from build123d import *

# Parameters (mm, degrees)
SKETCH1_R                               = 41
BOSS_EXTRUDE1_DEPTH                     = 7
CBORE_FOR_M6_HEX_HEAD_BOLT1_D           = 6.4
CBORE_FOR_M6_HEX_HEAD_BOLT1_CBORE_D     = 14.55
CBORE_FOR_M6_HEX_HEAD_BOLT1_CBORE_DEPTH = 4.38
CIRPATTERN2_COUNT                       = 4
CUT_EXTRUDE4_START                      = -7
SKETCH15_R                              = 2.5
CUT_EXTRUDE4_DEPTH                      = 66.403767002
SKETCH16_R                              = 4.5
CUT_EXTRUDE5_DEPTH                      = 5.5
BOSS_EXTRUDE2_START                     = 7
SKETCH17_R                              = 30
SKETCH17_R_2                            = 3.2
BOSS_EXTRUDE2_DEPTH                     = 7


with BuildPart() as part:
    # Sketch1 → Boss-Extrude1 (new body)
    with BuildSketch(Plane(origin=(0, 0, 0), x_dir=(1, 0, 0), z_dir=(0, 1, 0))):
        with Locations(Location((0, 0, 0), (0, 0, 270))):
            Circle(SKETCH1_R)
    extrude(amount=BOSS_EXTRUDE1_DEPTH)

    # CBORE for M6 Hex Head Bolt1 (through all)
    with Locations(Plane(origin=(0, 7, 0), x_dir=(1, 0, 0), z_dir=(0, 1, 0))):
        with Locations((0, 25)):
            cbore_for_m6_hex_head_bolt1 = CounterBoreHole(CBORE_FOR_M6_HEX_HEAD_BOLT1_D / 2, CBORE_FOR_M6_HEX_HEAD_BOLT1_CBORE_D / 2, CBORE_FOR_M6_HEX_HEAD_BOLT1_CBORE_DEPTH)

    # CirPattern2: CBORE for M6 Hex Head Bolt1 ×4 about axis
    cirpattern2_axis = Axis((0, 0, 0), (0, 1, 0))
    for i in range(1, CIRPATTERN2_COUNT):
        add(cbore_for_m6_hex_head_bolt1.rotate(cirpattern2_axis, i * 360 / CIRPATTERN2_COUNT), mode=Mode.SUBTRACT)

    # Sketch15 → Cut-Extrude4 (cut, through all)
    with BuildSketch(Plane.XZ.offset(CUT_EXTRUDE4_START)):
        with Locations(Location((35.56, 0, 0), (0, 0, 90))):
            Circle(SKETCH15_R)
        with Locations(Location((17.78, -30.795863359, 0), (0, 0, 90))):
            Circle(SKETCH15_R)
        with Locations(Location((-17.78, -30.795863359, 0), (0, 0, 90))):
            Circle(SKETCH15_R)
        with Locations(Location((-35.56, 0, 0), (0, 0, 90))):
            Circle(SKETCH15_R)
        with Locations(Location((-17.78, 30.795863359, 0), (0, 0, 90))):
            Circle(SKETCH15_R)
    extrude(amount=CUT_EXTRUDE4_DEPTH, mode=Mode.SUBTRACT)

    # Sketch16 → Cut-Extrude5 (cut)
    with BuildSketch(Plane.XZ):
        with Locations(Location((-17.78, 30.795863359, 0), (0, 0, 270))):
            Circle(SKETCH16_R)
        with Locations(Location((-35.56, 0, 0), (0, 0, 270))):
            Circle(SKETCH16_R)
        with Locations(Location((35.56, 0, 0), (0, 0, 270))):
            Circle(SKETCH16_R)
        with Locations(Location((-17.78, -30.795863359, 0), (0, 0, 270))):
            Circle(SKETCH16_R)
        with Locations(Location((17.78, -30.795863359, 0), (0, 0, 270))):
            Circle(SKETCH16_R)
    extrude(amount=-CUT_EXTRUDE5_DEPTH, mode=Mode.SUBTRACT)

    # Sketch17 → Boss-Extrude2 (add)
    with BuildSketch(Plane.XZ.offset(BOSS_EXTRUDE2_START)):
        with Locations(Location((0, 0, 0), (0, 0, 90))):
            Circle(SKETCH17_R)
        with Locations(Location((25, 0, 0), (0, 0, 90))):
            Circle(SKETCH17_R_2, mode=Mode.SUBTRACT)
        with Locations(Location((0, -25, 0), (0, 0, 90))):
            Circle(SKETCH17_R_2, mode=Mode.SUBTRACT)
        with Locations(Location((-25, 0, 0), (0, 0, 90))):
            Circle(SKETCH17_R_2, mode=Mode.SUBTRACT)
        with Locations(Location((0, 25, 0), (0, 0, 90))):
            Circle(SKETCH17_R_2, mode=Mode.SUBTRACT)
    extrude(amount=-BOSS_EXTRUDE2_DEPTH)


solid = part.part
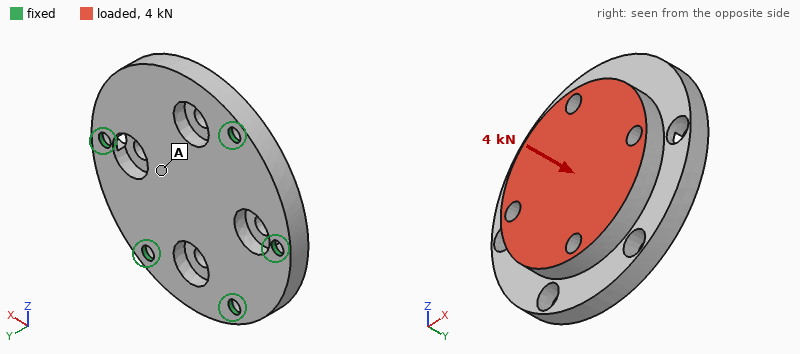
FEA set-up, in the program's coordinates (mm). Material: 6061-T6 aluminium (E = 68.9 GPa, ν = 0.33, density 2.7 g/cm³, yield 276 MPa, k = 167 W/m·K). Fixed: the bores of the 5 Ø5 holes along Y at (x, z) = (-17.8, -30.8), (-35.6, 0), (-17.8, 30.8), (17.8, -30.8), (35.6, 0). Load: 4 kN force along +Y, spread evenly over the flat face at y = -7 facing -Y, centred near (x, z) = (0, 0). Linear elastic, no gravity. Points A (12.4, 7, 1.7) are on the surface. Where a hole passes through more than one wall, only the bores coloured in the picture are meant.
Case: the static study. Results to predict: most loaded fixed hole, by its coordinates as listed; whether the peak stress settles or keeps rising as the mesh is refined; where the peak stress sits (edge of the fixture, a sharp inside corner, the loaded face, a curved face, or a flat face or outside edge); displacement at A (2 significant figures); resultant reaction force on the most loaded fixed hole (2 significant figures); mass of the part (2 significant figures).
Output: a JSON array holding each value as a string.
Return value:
["(-17.8, 30.8)", "keeps rising", "edge of the fixture", "22 µm", "1.7 kN", "140 g"]
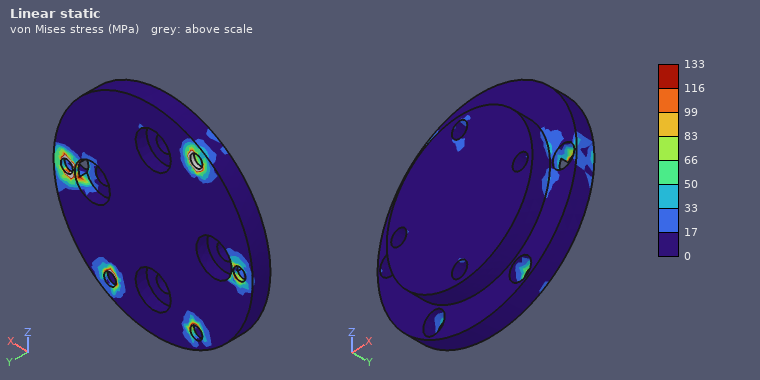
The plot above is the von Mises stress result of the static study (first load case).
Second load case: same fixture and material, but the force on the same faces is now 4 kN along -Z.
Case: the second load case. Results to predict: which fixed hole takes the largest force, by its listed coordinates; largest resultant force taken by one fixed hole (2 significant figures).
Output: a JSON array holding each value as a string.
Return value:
["(-17.8, 30.8)", "1.4 kN"]
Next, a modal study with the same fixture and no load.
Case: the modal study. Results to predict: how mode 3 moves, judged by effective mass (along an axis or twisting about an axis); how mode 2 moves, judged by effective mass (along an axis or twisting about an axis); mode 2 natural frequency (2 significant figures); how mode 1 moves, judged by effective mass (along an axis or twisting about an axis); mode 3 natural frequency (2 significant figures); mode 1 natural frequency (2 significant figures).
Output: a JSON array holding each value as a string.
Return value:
["along X", "along Y", "9900 Hz", "along Y", "11 kHz", "5800 Hz"]
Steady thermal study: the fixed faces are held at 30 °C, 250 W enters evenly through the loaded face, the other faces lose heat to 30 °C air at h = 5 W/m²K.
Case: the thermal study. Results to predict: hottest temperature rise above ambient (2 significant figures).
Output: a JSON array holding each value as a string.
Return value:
["62 K"]
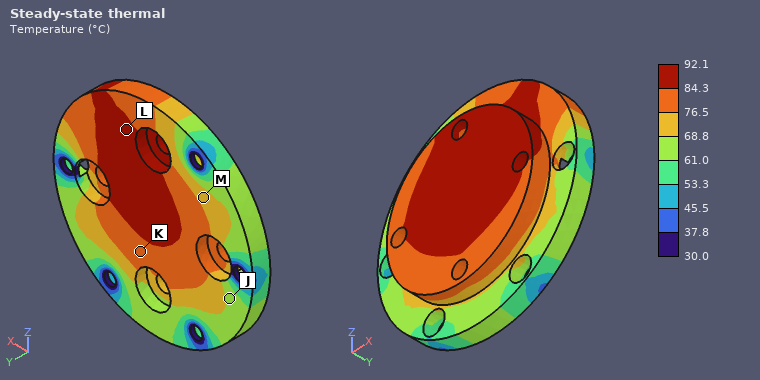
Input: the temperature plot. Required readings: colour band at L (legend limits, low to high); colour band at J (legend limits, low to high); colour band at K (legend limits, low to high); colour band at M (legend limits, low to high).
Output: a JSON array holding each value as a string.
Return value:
["84.3 to 92.1 °C", "61.0 to 68.8 °C", "76.5 to 84.3 °C", "68.8 to 76.5 °C"]
